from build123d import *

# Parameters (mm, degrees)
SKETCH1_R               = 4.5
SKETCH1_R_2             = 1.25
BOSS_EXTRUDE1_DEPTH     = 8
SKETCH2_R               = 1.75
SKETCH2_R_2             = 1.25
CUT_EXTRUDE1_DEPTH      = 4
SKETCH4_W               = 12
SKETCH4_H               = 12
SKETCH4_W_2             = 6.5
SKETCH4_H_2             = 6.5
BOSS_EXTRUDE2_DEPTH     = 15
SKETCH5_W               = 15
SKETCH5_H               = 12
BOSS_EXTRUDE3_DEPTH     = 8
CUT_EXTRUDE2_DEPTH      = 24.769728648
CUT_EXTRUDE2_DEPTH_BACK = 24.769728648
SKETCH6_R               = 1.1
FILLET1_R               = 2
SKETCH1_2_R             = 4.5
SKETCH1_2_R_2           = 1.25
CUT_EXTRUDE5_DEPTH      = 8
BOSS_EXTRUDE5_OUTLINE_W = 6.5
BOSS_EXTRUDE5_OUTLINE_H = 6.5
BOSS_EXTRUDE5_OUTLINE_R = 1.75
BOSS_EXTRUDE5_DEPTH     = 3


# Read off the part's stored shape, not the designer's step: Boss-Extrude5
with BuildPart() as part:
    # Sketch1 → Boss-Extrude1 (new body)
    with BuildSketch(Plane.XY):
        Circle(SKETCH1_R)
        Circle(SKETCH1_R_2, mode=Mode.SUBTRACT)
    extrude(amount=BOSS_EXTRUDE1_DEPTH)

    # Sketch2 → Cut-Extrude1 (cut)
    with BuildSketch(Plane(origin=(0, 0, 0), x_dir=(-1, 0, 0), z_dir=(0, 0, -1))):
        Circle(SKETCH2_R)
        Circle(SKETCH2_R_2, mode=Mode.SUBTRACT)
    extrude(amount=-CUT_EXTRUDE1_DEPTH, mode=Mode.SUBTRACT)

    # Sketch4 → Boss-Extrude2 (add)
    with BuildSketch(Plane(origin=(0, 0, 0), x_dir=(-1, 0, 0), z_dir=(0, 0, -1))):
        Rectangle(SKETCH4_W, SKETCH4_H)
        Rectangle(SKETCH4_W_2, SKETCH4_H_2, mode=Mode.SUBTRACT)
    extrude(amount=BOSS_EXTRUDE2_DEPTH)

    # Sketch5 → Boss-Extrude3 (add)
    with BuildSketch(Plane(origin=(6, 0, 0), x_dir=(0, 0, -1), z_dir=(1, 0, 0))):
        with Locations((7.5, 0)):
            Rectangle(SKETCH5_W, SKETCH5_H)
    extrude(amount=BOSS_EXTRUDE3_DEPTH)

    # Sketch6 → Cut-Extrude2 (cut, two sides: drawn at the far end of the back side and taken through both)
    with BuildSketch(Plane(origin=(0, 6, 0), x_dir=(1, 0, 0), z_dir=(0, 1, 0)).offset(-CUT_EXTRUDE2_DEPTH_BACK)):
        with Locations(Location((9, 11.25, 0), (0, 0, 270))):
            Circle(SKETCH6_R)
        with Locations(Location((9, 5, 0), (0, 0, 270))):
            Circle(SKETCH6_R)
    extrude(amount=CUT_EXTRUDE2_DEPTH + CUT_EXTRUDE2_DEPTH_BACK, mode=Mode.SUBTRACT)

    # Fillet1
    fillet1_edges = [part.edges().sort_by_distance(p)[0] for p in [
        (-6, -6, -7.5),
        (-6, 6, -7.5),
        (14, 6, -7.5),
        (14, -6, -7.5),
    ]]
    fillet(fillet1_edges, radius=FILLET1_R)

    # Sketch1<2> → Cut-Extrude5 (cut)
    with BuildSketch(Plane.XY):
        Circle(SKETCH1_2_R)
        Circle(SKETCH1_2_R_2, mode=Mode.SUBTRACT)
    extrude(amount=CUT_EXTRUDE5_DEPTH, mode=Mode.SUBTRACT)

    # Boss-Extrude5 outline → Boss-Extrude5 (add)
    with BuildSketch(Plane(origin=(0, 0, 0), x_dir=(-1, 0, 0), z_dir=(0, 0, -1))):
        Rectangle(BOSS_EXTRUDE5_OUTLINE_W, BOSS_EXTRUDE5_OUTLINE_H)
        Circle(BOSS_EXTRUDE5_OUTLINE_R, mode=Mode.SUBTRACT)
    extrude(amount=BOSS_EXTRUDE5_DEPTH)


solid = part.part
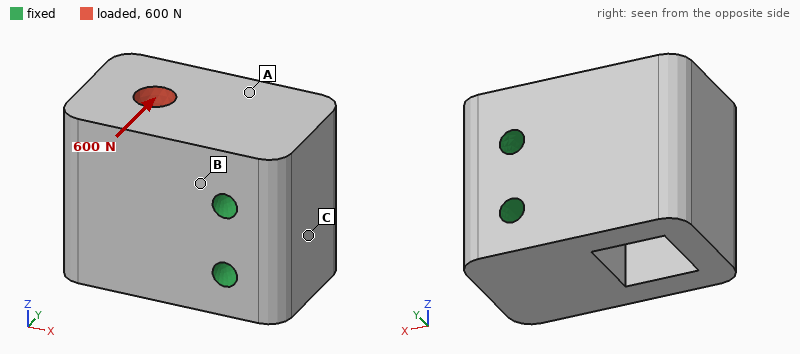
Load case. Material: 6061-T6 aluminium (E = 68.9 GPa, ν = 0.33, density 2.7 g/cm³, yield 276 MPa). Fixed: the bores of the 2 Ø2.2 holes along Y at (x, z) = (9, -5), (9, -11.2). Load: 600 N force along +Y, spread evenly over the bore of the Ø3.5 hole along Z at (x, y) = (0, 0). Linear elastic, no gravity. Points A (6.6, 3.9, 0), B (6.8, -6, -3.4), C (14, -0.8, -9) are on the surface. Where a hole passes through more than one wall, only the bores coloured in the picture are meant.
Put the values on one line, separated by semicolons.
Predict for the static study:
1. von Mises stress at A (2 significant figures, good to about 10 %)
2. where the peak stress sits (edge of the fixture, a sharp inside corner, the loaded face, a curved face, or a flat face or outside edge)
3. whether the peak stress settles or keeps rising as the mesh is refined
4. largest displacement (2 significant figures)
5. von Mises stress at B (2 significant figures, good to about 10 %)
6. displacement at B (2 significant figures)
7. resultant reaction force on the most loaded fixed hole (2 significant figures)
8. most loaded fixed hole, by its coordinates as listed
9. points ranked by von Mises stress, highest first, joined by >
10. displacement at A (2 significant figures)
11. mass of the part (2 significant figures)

9.8 MPa; edge of the fixture; keeps rising; 8.5 µm; 27 MPa; 1.4 µm; 540 N; (9, -5); B > A > C; 1.6 µm; 7.9 g
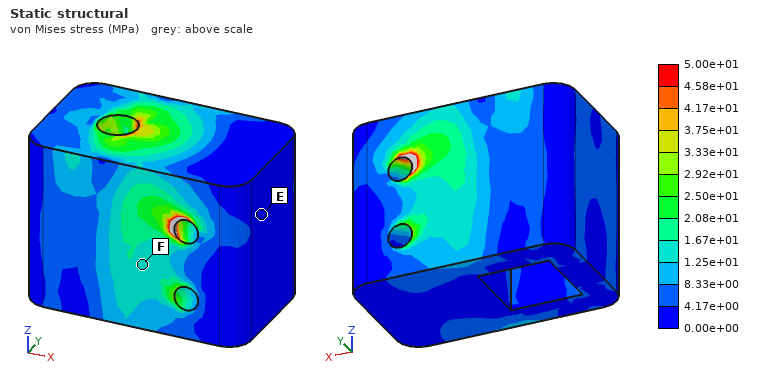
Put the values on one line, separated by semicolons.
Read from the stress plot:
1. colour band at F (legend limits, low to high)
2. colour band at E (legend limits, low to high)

1.25e+01 to 1.67e+01 MPa; 0.00e+00 to 4.17e+00 MPa
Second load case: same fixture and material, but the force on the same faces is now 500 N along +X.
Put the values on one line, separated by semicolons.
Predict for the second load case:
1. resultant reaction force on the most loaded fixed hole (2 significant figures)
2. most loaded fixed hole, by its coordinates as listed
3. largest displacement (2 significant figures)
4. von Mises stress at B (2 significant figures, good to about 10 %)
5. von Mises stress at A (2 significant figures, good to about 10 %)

670 N; (9, -5); 3.7 µm; 11 MPa; 7.3 MPa
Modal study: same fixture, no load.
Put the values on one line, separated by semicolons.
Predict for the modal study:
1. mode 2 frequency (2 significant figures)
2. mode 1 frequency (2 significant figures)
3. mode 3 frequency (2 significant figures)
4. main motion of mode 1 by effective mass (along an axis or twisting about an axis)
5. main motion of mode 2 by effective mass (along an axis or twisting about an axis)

29 kHz; 24 kHz; 43 kHz; along Y; along Z
